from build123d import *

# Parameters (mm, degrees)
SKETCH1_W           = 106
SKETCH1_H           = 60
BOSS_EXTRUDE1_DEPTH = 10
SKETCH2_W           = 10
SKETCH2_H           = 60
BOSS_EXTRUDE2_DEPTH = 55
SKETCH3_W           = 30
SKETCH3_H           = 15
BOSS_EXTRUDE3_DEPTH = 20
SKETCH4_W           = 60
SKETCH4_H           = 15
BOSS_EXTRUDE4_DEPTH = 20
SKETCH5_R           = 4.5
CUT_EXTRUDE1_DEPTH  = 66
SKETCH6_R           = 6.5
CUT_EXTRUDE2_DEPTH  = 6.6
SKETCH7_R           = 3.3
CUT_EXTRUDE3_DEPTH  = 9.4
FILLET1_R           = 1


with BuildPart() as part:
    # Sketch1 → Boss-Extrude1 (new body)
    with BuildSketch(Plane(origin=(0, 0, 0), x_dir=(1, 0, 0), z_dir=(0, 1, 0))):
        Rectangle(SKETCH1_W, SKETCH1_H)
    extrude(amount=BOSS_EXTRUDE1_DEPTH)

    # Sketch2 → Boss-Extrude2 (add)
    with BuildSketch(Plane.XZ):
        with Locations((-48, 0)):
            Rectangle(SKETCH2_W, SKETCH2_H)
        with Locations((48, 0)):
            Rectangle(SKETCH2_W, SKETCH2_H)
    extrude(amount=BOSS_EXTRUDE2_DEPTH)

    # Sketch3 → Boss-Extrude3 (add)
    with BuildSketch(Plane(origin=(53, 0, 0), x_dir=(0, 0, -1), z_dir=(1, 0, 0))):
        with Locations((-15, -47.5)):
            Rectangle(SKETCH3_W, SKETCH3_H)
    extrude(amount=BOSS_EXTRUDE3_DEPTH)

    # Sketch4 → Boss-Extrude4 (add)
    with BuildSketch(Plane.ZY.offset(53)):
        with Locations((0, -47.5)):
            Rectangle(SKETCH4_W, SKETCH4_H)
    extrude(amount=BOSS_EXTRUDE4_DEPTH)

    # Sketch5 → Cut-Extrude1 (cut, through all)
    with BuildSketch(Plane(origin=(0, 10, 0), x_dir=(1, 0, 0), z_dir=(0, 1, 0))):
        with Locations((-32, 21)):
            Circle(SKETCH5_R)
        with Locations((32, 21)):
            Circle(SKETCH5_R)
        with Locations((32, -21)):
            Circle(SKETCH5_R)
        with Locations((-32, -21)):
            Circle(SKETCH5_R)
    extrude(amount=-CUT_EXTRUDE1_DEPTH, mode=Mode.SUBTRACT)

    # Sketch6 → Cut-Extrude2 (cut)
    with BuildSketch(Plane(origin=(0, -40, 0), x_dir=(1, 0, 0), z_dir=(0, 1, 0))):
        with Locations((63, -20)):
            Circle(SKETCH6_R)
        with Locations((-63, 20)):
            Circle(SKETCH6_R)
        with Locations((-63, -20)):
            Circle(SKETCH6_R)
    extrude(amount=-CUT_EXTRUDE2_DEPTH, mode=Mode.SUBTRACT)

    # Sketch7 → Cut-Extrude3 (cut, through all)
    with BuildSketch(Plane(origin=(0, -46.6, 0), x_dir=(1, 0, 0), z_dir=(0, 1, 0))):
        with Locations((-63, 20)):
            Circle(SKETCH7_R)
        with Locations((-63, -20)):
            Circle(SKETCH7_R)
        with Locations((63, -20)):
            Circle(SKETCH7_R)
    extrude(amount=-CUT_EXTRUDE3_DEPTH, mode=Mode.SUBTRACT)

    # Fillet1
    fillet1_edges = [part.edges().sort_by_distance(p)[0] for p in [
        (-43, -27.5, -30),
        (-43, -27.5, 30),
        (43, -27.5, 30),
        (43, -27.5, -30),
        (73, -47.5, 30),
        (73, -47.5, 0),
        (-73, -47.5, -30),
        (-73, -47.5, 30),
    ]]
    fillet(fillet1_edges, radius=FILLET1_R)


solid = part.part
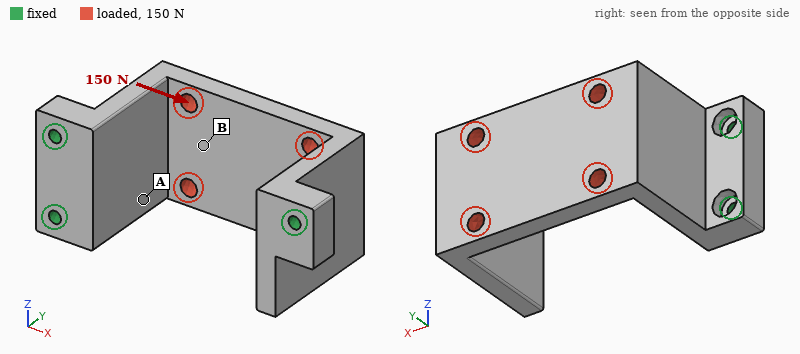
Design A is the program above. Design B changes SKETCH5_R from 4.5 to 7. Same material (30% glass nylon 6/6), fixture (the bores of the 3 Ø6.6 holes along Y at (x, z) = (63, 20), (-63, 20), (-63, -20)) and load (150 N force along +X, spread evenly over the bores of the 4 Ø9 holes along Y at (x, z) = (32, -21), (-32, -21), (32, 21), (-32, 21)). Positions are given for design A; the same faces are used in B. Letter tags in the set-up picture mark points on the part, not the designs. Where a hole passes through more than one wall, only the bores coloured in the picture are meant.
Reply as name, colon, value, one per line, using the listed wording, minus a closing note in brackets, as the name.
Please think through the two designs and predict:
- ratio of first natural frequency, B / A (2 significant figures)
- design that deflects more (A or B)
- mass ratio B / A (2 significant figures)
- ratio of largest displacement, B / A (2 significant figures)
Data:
ratio of first natural frequency, B / A: 1.0
design that deflects more: B
mass ratio B / A: 0.98
ratio of largest displacement, B / A: 1.1
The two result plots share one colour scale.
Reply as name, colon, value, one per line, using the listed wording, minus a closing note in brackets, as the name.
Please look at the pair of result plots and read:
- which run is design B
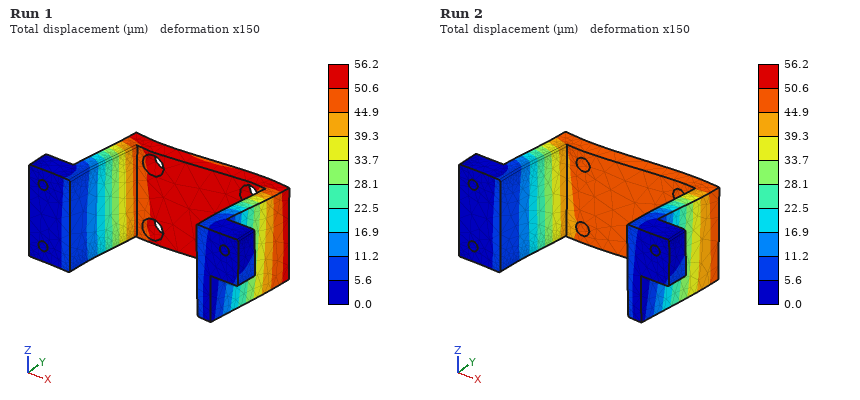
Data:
which run is design B: Run 1
